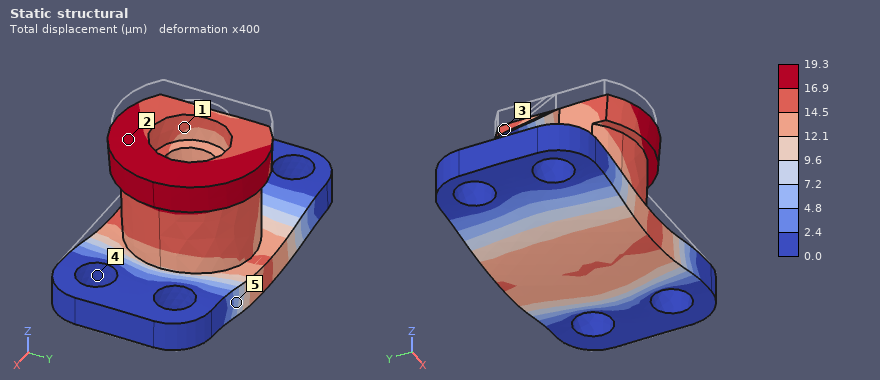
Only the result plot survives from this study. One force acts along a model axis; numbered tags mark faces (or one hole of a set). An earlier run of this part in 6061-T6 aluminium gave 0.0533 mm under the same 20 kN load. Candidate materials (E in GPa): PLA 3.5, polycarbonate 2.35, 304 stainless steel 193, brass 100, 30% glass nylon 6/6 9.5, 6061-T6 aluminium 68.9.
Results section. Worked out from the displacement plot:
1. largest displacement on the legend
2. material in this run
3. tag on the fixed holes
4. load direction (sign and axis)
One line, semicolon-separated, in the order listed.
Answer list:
19.3 µm; 304 stainless steel; 4; -Z
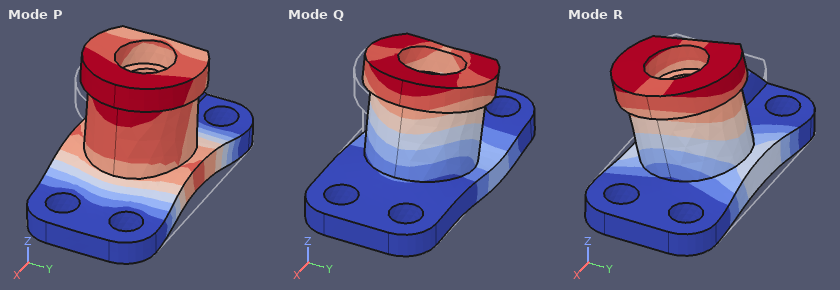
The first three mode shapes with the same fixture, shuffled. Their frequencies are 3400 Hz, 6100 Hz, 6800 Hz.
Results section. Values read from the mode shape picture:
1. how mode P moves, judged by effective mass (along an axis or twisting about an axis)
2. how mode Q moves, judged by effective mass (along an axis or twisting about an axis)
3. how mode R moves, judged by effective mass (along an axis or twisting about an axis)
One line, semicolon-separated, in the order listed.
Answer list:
along Z; along X; along Y
